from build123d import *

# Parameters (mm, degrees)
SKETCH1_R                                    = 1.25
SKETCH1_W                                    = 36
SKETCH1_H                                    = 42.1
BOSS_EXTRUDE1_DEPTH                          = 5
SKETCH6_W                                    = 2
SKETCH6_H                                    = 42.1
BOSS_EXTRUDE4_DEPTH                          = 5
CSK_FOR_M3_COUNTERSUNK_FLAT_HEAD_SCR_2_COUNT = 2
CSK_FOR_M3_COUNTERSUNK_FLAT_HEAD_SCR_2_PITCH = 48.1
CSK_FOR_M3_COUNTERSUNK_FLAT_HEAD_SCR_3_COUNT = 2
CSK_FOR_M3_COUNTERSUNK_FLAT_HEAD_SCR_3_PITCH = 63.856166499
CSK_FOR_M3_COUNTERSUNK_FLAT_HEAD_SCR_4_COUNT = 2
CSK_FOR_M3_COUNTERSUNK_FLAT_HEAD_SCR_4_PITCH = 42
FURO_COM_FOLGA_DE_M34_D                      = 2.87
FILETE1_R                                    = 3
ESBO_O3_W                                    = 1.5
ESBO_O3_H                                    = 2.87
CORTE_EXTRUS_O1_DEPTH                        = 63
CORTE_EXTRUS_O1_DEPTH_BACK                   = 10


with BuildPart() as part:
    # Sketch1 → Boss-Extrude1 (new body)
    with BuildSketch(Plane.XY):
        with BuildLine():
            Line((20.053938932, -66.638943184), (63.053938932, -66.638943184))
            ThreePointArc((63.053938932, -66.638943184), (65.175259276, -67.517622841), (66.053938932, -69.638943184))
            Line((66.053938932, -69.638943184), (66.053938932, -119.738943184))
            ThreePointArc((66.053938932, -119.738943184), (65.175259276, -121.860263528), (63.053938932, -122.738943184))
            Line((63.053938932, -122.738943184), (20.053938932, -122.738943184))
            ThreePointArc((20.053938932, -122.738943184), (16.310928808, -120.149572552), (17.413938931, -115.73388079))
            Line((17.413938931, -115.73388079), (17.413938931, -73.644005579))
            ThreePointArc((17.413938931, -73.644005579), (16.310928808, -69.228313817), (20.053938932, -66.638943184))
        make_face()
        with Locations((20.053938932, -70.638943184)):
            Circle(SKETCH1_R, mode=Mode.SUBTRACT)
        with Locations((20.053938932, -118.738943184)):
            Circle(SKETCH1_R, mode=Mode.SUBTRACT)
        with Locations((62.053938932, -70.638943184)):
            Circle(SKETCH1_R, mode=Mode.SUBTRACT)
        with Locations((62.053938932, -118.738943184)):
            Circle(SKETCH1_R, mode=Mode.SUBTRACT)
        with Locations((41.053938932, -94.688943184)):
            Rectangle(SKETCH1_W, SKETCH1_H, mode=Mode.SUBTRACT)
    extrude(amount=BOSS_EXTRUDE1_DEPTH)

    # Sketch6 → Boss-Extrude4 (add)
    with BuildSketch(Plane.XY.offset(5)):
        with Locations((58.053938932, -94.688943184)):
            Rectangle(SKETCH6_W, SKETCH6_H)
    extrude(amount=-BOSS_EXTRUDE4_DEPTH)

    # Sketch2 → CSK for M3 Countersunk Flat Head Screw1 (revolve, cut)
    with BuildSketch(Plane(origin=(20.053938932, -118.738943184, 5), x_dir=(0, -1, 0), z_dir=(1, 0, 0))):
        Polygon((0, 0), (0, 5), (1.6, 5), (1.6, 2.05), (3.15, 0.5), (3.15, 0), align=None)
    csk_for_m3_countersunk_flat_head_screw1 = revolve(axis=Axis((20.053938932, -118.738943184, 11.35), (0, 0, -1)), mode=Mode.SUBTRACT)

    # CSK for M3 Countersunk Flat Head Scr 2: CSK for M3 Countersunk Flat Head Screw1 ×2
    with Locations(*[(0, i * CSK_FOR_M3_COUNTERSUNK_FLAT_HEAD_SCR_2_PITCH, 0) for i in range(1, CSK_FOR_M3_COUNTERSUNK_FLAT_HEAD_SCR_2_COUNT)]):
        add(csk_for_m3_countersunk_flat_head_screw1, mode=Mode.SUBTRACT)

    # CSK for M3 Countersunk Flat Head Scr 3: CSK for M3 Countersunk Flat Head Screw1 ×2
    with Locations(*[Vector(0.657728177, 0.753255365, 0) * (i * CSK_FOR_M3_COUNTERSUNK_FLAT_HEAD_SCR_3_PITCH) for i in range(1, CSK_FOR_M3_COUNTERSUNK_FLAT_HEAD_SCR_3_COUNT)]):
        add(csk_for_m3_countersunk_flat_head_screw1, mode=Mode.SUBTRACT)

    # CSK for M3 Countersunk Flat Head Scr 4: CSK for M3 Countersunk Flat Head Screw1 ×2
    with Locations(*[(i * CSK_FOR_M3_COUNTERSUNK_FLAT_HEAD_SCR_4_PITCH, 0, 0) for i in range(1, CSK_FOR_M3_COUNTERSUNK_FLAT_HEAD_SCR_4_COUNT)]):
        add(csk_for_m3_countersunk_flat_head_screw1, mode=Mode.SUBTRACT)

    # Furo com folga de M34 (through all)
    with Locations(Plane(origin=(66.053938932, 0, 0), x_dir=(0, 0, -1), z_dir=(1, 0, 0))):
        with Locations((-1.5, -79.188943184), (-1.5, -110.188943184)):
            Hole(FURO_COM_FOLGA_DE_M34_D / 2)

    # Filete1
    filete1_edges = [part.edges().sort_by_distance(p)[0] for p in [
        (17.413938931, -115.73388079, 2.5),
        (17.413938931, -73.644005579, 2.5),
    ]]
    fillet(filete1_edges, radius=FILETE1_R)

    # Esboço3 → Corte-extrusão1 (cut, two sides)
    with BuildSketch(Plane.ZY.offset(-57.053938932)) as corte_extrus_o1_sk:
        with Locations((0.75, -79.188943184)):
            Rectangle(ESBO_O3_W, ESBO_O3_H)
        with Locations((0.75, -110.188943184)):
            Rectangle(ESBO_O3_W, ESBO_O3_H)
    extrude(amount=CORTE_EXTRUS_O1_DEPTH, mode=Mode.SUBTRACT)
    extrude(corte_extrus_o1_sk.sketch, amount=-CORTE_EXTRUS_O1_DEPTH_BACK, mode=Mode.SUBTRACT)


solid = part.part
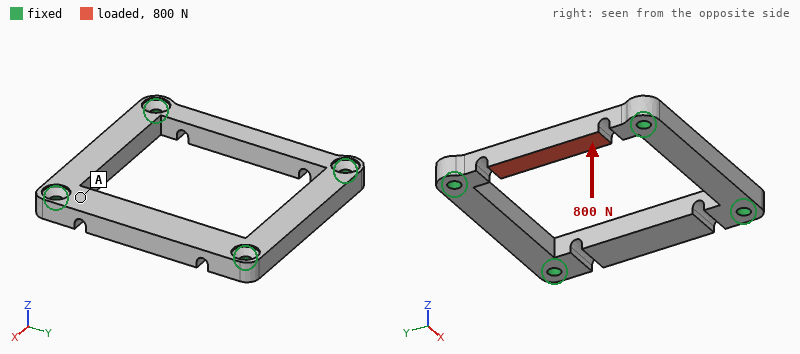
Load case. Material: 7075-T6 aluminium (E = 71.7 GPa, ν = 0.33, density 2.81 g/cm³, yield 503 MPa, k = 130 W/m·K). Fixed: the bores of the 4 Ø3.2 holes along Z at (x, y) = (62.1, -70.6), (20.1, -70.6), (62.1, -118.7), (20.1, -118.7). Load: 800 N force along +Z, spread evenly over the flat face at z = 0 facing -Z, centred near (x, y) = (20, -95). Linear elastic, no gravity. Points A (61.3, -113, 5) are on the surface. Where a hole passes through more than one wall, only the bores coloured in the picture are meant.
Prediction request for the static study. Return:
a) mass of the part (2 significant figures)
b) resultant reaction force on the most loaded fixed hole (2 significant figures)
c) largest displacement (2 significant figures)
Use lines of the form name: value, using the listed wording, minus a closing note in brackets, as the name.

mass of the part: 17 g
resultant reaction force on the most loaded fixed hole: 410 N
largest displacement: 0.12 mm
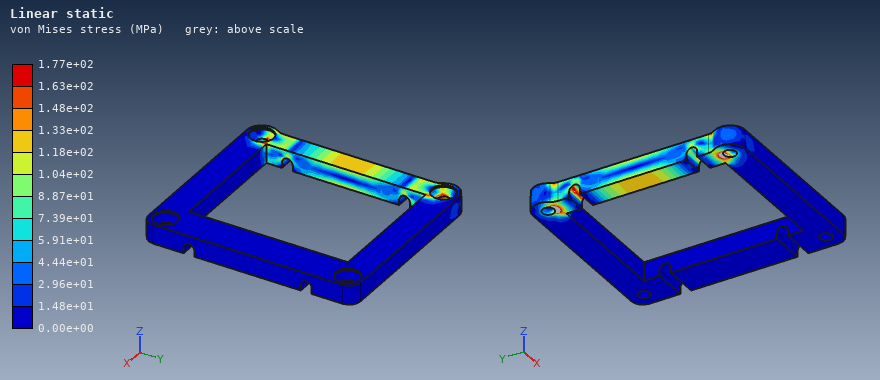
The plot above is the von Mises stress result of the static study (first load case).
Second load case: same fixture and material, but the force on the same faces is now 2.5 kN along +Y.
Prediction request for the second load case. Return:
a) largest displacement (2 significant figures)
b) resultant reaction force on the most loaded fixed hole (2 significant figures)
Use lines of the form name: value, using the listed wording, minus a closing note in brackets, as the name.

largest displacement: 51 µm
resultant reaction force on the most loaded fixed hole: 1.3 kN
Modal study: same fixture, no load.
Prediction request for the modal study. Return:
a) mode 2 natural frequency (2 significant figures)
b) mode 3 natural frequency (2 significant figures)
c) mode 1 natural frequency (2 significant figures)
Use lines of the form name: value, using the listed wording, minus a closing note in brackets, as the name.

mode 2 natural frequency: 9400 Hz
mode 3 natural frequency: 11 kHz
mode 1 natural frequency: 9100 Hz
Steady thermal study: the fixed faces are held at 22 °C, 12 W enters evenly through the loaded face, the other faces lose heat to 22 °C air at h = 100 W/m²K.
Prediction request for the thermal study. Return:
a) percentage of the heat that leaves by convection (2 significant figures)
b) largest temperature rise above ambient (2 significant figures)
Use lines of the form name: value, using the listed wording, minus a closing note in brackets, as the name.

percentage of the heat that leaves by convection: 14 %
largest temperature rise above ambient: 33 K
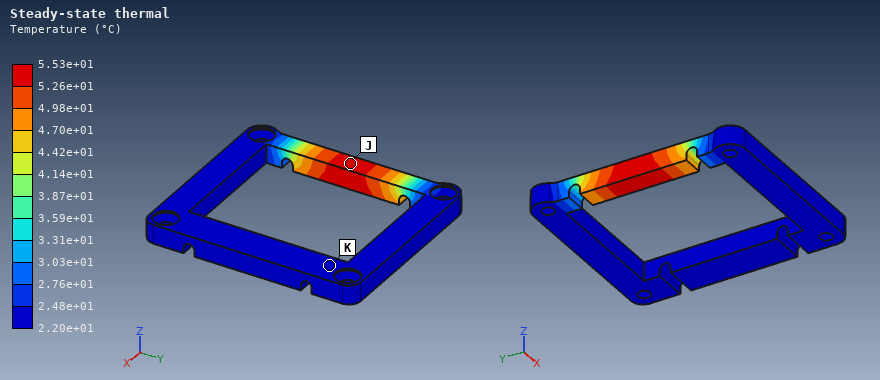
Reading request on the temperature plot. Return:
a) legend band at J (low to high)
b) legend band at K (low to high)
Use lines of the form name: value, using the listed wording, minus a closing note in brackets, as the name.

legend band at J: 5.26e+01 to 5.53e+01 °C
legend band at K: 2.20e+01 to 2.48e+01 °C
